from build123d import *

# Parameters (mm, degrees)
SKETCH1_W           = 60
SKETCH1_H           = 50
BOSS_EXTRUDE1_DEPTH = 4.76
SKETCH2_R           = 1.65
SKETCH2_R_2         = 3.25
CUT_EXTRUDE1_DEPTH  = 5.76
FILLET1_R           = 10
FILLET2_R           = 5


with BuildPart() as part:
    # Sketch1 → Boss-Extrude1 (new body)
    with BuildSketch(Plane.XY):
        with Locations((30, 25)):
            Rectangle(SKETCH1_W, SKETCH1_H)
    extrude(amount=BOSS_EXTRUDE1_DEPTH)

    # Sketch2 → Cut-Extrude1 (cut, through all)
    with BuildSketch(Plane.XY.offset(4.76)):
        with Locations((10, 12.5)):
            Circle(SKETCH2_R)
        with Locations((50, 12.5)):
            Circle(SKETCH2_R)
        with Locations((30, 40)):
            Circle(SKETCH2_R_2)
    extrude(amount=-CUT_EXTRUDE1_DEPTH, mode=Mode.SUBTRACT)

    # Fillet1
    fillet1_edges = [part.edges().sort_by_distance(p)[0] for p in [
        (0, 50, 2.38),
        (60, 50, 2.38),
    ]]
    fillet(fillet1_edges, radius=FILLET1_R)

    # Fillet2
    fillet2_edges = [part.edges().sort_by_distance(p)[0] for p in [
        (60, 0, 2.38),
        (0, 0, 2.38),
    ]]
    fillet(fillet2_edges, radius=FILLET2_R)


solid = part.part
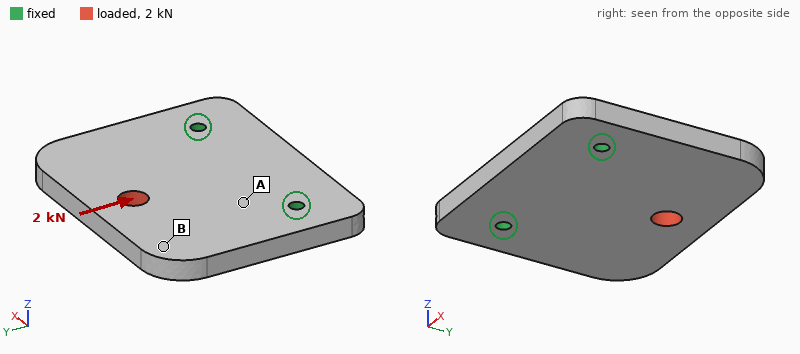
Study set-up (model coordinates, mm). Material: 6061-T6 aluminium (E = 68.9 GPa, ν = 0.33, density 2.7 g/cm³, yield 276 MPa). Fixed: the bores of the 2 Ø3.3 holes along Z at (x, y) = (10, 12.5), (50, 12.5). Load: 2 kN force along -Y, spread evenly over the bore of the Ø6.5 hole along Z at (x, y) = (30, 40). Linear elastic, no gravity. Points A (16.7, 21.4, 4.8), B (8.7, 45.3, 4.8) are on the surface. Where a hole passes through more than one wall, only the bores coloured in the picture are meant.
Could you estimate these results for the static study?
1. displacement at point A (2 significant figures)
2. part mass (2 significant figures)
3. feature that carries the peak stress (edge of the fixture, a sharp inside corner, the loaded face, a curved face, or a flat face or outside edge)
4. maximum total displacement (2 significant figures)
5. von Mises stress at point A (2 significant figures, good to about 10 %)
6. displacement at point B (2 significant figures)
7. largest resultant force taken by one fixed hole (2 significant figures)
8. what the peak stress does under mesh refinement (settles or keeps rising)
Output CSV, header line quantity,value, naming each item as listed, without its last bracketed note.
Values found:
quantity,value
displacement at point A,2.7 µm
part mass,37 g
feature that carries the peak stress,edge of the fixture
maximum total displacement,9.9 µm
von Mises stress at point A,13 MPa
displacement at point B,2.9 µm
largest resultant force taken by one fixed hole,1.0 kN
what the peak stress does under mesh refinement,keeps rising
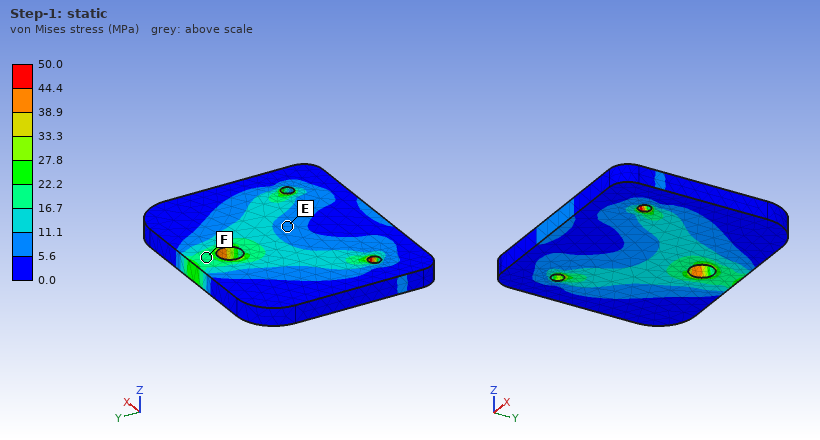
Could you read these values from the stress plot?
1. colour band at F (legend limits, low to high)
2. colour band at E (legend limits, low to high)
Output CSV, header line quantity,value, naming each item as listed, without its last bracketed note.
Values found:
quantity,value
colour band at F,16.7 to 22.2 MPa
colour band at E,5.6 to 11.1 MPa
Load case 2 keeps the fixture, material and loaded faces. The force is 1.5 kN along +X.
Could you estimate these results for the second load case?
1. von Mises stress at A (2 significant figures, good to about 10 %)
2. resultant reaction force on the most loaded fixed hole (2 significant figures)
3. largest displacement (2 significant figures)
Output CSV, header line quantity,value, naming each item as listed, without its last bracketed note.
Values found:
quantity,value
von Mises stress at A,14 MPa
resultant reaction force on the most loaded fixed hole,1.2 kN
largest displacement,13 µm
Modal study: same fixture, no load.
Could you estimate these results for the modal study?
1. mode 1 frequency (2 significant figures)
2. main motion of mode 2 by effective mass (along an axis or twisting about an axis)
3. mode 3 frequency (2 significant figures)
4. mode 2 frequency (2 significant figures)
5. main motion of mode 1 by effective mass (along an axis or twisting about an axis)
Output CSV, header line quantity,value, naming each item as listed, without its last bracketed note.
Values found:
quantity,value
mode 1 frequency,2500 Hz
main motion of mode 2 by effective mass,twisting about Y
mode 3 frequency,9500 Hz
mode 2 frequency,4800 Hz
main motion of mode 1 by effective mass,along Z
